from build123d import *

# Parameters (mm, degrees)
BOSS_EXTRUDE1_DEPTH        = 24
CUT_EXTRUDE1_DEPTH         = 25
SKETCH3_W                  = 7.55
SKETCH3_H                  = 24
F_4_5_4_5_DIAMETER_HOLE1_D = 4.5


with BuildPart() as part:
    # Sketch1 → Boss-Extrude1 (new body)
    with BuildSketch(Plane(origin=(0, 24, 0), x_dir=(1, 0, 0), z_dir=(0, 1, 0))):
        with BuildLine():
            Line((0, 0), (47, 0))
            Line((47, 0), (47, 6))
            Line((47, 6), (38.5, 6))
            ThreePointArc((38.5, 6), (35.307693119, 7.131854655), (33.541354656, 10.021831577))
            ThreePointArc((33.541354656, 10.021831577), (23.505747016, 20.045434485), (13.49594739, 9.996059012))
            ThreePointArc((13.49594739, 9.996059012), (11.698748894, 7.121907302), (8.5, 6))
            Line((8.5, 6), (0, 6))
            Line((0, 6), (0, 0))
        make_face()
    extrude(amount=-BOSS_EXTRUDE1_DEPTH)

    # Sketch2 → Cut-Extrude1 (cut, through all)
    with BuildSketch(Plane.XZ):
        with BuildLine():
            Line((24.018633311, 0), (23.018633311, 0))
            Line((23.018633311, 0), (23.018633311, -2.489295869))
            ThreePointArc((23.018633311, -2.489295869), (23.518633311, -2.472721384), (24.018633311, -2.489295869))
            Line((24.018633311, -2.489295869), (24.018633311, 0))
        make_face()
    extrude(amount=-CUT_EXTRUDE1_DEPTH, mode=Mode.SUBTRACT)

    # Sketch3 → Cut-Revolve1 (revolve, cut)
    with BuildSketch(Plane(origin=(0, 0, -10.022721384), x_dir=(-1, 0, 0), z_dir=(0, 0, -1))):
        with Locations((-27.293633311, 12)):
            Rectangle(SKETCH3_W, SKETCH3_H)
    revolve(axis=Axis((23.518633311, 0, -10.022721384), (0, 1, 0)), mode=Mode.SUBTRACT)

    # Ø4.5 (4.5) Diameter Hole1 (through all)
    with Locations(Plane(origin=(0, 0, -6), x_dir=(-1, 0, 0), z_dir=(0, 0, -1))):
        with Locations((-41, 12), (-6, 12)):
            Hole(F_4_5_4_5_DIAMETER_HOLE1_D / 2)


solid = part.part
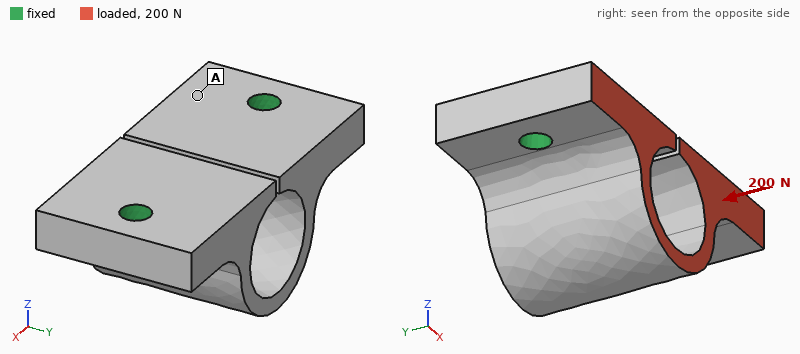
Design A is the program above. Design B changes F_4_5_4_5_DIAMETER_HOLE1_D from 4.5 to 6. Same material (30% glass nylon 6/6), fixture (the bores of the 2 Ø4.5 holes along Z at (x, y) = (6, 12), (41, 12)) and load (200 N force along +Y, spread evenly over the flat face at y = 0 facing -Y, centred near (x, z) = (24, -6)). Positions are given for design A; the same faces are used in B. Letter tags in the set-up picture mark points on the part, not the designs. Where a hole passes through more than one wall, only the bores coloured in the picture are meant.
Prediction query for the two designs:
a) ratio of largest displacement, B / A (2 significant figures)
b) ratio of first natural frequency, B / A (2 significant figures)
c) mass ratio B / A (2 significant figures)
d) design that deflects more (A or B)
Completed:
0.72
1.2
0.98
A
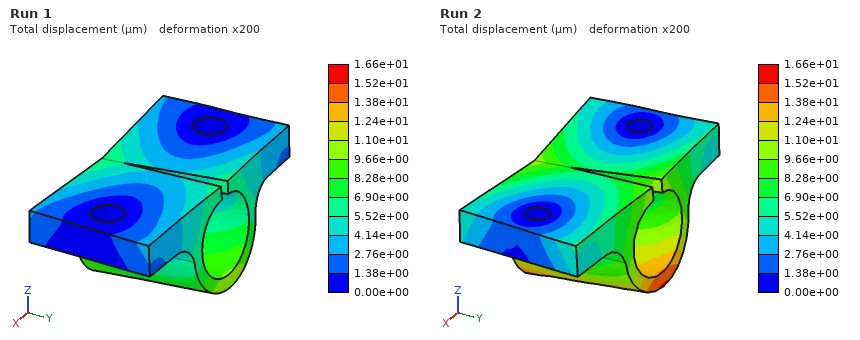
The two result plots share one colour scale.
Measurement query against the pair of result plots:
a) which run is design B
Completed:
Run 1
